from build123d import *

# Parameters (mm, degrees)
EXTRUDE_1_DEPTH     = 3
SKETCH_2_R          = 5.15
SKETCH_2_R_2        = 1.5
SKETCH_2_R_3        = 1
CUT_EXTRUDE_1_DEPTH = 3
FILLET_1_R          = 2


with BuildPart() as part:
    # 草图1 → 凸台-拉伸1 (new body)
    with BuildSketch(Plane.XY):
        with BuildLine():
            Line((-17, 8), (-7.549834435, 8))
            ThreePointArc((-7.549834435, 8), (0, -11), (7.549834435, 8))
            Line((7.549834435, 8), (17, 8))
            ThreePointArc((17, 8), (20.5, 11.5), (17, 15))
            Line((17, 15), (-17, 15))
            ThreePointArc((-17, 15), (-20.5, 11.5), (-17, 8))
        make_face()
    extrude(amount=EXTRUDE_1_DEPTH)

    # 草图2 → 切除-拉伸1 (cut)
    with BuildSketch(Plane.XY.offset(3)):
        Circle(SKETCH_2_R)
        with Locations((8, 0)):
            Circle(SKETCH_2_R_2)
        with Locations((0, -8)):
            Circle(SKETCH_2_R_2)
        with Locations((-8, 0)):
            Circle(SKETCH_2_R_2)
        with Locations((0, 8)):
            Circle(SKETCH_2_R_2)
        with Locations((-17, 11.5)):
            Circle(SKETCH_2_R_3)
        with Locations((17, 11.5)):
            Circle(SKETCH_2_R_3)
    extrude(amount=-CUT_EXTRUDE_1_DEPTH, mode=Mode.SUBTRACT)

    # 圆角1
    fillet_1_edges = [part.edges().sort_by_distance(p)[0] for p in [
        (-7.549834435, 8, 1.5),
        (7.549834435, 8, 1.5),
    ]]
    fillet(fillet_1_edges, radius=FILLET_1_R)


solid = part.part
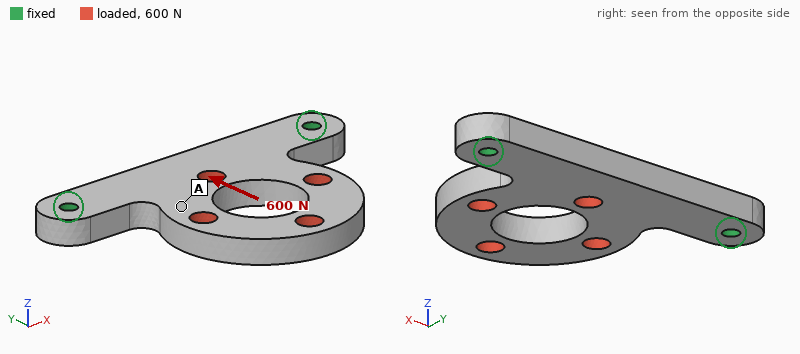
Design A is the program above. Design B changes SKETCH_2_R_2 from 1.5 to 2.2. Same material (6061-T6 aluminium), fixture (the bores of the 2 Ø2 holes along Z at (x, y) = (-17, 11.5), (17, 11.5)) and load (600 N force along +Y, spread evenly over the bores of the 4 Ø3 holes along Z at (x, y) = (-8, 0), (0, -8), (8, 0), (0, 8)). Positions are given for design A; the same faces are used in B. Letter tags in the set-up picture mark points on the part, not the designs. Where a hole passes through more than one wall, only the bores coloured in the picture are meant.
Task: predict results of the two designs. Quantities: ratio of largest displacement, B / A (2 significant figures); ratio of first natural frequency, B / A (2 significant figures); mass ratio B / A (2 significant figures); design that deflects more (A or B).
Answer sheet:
1.2
1.0
0.94
B
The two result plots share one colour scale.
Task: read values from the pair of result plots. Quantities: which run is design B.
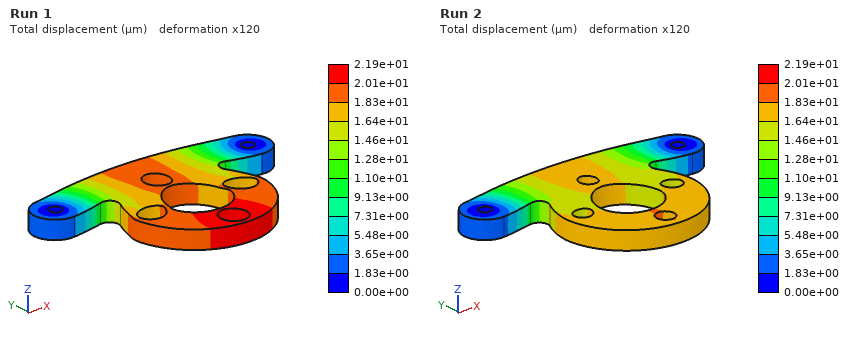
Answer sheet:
Run 1
